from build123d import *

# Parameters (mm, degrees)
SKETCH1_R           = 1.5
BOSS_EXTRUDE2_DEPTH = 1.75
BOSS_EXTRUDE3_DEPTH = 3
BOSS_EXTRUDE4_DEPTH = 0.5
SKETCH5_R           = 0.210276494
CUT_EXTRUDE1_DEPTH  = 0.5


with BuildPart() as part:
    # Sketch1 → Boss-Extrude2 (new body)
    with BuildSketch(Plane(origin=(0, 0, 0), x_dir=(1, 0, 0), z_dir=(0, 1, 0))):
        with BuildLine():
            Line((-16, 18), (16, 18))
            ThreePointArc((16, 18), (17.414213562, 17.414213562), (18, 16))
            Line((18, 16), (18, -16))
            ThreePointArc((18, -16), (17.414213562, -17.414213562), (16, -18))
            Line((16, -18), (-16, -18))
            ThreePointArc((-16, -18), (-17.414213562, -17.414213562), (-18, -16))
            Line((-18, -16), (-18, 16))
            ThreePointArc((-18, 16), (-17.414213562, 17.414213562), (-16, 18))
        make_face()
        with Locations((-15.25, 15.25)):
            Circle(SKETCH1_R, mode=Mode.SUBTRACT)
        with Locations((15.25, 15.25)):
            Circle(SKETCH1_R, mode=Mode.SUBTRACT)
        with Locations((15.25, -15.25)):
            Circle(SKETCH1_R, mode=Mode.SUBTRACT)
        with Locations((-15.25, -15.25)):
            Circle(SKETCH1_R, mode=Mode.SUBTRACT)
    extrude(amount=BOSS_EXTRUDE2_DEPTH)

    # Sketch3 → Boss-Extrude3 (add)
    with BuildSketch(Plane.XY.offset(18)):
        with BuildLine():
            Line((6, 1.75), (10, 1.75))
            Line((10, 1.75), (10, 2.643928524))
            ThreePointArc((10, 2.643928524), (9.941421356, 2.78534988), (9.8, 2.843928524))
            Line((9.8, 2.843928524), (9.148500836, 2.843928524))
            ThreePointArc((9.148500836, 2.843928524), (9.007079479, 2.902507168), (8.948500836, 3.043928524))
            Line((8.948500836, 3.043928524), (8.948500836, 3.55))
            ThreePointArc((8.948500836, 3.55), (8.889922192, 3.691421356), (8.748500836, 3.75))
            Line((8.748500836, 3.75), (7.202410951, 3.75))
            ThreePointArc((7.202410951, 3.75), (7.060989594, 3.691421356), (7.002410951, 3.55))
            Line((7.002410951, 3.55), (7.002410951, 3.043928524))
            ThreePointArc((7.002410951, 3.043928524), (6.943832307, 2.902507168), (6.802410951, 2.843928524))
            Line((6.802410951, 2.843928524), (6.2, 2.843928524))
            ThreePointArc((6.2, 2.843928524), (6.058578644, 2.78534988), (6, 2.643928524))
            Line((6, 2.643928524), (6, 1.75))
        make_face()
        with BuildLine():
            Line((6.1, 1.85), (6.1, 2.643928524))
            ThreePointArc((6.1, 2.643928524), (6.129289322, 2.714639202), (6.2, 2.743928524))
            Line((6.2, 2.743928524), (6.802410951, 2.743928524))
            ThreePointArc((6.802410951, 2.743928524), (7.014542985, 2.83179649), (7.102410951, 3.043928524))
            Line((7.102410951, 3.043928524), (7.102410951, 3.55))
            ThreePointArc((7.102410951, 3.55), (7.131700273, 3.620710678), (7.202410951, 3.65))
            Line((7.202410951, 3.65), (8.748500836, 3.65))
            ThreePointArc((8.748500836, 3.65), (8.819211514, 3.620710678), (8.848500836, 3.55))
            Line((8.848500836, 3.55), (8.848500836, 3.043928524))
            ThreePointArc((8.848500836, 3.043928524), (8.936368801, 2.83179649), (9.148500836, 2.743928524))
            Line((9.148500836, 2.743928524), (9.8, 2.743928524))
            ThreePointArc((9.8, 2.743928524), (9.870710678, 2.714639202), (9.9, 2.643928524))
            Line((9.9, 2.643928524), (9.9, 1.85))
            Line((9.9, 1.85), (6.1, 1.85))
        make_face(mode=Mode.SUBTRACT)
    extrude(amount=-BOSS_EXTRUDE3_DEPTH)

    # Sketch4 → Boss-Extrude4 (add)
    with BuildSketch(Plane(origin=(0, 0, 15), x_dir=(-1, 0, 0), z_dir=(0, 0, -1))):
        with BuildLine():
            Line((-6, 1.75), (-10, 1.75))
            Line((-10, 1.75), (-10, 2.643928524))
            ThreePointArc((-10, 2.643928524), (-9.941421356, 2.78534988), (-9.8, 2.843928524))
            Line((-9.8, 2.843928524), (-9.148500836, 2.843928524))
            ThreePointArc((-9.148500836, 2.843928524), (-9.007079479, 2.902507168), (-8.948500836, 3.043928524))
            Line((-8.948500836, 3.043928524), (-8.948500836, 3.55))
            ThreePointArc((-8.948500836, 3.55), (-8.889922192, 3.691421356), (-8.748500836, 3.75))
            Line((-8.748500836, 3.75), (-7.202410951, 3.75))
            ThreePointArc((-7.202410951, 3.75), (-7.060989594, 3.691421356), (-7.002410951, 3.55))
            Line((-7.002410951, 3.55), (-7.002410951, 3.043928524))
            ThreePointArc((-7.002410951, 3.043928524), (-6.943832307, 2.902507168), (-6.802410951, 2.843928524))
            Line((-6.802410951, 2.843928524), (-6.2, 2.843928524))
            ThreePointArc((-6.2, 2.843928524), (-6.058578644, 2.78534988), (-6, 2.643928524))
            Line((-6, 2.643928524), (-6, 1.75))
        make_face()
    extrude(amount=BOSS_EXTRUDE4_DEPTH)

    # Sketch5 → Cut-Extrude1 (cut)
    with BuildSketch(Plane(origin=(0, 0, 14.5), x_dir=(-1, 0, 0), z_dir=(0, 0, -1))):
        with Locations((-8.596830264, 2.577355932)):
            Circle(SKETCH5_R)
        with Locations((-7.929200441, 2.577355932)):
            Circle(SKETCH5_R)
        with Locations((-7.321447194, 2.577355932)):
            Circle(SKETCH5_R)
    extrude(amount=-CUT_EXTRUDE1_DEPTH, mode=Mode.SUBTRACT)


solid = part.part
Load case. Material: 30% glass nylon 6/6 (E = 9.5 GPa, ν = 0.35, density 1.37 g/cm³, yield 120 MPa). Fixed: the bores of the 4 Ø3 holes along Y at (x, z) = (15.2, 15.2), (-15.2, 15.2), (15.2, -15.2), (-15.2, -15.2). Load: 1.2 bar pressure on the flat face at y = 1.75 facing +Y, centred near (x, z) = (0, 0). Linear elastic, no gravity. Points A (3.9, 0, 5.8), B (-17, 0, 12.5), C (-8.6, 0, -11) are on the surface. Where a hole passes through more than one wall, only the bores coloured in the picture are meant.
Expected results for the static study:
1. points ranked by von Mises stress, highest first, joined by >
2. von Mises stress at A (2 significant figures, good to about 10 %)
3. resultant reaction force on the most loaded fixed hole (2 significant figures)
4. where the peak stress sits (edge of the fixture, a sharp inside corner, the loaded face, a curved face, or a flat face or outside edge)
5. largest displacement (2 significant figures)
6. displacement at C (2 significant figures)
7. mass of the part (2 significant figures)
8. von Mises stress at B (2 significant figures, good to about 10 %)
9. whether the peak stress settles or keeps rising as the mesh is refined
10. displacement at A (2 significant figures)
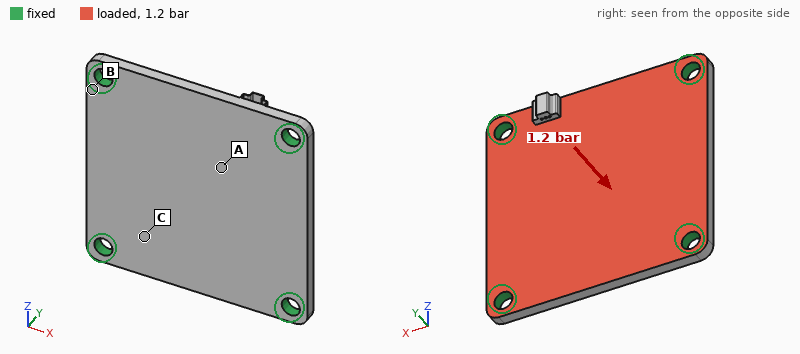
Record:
B > A > C
9.3 MPa
38 N
edge of the fixture
0.14 mm
0.059 mm
3.0 g
15 MPa
keeps rising
0.12 mm
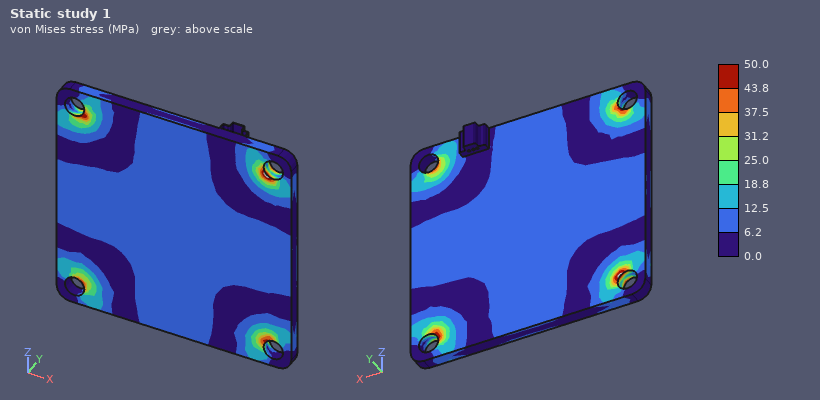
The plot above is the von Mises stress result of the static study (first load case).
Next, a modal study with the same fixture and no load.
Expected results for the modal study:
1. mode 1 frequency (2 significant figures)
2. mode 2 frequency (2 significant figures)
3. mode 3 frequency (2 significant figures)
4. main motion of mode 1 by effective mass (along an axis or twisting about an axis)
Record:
3700 Hz
6100 Hz
6200 Hz
along Y
